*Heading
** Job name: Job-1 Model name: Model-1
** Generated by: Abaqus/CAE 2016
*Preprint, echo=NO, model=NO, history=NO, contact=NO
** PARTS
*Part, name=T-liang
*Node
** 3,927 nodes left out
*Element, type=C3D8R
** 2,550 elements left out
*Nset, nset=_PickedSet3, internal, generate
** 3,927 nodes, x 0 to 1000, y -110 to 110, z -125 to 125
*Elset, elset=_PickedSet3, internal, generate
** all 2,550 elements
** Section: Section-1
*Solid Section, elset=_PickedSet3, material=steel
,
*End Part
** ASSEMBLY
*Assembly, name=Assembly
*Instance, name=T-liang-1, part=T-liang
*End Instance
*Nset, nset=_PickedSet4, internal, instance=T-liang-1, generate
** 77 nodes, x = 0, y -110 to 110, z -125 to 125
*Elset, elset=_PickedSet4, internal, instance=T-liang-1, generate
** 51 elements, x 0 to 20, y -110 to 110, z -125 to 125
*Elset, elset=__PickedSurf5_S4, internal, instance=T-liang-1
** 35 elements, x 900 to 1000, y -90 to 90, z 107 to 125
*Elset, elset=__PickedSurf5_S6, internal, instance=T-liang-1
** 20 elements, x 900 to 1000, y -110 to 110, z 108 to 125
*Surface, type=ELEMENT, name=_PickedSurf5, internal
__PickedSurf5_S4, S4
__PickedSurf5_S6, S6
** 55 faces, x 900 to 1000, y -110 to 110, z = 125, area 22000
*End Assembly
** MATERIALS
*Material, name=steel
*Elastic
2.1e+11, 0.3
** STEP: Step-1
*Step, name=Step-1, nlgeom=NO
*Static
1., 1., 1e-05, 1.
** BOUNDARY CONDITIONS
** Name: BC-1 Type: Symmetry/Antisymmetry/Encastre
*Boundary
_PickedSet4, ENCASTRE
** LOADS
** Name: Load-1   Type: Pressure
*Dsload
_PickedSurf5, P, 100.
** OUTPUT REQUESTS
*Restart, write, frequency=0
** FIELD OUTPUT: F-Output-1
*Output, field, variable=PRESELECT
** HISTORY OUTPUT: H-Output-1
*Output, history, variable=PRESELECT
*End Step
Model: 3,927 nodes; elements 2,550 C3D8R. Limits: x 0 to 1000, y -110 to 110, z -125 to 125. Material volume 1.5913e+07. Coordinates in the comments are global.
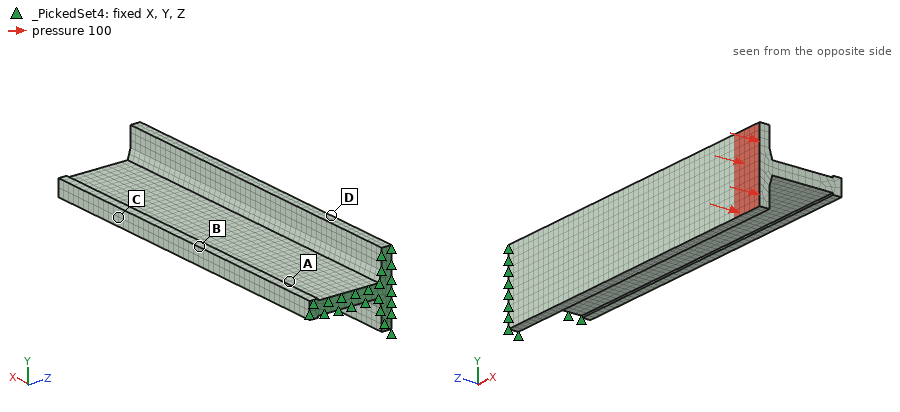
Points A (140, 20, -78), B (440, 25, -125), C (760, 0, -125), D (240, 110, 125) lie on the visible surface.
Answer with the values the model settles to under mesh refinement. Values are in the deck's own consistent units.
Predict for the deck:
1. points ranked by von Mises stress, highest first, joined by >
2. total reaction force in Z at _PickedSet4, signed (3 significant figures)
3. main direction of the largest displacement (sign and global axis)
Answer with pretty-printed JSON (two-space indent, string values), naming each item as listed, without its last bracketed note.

{
  "points ranked by von Mises stress, highest first, joined by >": "A > B > D > C",
  "total reaction force in Z at _PickedSet4, signed": "2.20e+06",
  "main direction of the largest displacement": "-Z"
}
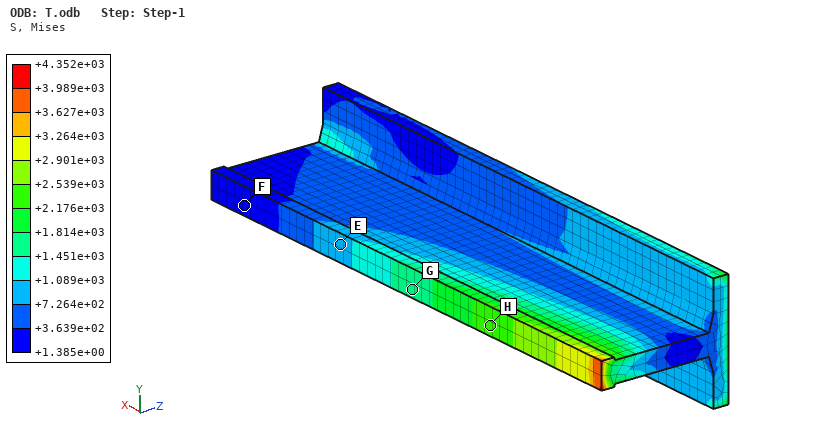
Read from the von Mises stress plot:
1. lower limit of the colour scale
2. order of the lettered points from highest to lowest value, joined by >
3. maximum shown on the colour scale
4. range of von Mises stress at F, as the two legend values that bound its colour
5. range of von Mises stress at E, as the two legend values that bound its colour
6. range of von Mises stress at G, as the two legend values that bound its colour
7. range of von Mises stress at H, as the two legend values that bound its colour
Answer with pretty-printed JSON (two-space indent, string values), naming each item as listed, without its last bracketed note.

{
  "lower limit of the colour scale": "+1.385e+00",
  "order of the lettered points from highest to lowest value, joined by >": "H > G > E > F",
  "maximum shown on the colour scale": "+4.352e+03",
  "range of von Mises stress at F, as the two legend values that bound its colour": "+1.385e+00 to +3.639e+02",
  "range of von Mises stress at E, as the two legend values that bound its colour": "+7.264e+02 to +1.089e+03",
  "range of von Mises stress at G, as the two legend values that bound its colour": "+1.451e+03 to +1.814e+03",
  "range of von Mises stress at H, as the two legend values that bound its colour": "+2.176e+03 to +2.539e+03"
}
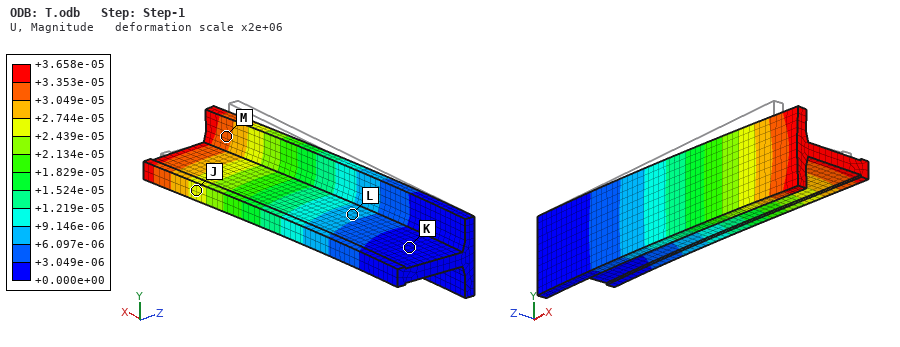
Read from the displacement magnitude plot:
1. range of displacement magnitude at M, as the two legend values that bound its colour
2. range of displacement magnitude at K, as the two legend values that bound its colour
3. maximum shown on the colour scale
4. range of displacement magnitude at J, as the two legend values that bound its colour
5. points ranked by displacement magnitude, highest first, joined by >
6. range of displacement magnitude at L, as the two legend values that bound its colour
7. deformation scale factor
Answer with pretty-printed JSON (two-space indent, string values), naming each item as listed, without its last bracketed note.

{
  "range of displacement magnitude at M, as the two legend values that bound its colour": "+3.049e-05 to +3.353e-05",
  "range of displacement magnitude at K, as the two legend values that bound its colour": "+0.000e+00 to +3.049e-06",
  "maximum shown on the colour scale": "+3.658e-05",
  "range of displacement magnitude at J, as the two legend values that bound its colour": "+2.439e-05 to +2.744e-05",
  "points ranked by displacement magnitude, highest first, joined by >": "M > J > L > K",
  "range of displacement magnitude at L, as the two legend values that bound its colour": "+6.097e-06 to +9.146e-06",
  "deformation scale factor": "2e+06"
}
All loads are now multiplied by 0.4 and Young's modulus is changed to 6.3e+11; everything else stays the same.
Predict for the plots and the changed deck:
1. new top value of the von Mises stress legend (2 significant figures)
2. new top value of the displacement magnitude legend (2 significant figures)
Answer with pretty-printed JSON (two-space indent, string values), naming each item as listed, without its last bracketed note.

{
  "new top value of the von Mises stress legend": "1700",
  "new top value of the displacement magnitude legend": "4.9e-06"
}
